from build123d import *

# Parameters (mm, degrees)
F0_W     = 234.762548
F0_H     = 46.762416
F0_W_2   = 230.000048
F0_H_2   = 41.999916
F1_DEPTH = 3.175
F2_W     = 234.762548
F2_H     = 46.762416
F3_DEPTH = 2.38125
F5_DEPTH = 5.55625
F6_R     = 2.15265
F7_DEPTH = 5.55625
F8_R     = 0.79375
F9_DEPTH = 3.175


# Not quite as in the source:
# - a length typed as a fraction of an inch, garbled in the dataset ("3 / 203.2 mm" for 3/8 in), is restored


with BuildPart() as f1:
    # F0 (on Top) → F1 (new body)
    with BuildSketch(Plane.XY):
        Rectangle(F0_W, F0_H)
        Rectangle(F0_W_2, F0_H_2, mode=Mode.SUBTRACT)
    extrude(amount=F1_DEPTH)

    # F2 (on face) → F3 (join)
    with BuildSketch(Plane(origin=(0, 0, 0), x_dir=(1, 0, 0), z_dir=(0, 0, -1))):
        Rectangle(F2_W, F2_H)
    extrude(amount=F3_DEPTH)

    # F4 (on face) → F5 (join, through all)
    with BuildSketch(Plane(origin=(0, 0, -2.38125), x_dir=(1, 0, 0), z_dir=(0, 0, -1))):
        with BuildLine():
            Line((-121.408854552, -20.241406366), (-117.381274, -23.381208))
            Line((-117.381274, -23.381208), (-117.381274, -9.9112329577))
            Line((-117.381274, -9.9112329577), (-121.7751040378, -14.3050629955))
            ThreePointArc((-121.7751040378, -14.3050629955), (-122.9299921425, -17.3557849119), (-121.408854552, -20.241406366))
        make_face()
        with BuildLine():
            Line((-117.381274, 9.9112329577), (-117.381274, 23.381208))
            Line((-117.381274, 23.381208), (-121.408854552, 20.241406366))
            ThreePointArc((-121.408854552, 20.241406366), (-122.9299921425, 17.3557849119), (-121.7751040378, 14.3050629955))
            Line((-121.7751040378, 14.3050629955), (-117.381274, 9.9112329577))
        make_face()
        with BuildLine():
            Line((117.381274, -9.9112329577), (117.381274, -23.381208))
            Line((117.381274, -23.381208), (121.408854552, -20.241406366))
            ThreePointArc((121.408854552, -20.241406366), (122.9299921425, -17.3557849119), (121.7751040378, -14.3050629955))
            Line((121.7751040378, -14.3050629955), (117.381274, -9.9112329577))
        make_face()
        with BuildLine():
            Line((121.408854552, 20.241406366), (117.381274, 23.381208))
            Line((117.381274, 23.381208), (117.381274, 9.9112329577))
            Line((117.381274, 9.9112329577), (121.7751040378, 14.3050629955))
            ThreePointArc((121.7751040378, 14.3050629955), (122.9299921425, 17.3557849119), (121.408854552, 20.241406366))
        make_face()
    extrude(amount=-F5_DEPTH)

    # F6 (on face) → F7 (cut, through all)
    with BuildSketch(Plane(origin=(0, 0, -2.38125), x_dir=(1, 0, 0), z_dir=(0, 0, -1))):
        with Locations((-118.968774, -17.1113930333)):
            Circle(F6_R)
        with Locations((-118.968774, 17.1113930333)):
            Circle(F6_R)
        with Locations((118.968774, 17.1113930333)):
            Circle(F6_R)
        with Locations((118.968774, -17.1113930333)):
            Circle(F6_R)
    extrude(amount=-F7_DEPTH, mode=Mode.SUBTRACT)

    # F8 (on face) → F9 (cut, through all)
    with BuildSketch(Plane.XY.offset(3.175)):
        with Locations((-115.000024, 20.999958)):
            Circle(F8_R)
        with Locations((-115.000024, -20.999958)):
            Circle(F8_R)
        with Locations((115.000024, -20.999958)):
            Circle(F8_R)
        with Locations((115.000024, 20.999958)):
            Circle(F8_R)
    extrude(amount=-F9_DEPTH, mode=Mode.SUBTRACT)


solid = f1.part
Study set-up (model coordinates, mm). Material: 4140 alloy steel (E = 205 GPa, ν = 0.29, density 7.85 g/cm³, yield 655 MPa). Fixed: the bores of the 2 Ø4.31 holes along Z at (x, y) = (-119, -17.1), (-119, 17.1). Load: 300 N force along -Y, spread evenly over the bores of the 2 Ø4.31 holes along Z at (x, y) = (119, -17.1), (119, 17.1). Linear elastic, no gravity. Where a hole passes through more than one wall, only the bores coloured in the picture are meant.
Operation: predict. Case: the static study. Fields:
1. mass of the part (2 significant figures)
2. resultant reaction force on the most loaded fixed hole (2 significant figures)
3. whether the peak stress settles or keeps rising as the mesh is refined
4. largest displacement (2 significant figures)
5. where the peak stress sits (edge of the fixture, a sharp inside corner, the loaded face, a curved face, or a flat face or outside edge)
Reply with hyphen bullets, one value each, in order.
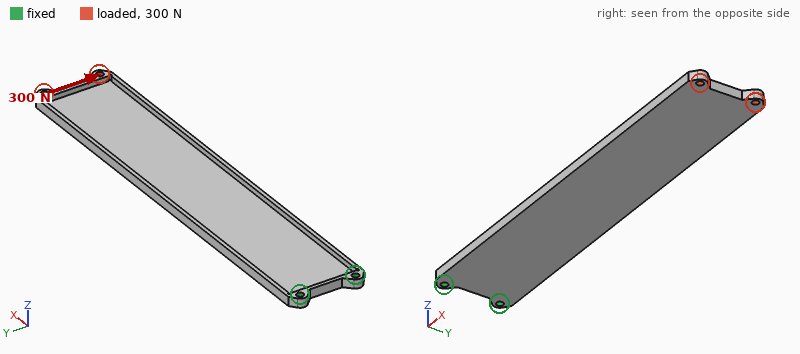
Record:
- 240 g
- 2.0 kN
- keeps rising
- 0.34 mm
- edge of the fixture
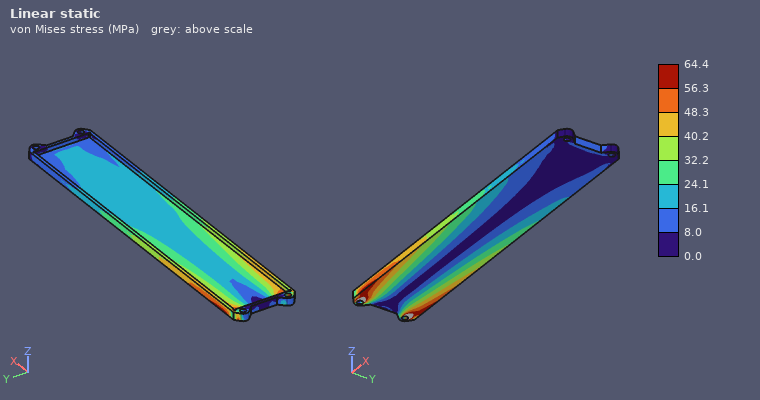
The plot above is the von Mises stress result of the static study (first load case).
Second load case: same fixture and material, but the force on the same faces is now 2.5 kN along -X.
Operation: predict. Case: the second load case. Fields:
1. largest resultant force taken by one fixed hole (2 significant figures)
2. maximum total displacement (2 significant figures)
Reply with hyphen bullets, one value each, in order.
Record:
- 1.3 kN
- 2.7 mm
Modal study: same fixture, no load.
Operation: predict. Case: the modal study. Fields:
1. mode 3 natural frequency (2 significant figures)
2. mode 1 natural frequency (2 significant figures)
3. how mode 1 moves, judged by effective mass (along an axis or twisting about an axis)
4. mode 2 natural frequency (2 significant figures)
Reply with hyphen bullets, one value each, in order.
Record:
- 350 Hz
- 56 Hz
- along Z
- 340 Hz
